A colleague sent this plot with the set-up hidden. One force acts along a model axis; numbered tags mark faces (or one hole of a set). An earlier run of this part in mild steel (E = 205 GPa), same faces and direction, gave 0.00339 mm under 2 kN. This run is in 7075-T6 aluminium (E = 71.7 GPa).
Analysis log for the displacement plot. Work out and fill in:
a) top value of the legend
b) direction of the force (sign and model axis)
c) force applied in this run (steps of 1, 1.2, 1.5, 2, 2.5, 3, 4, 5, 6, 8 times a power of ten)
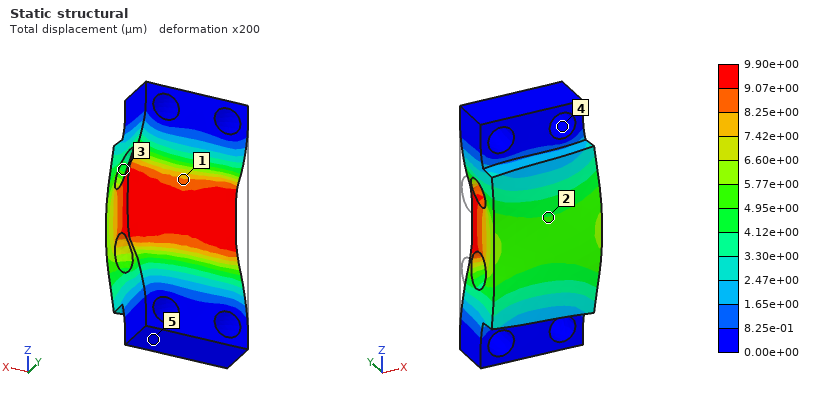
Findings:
9.90e+00 µm
+X
2 kN
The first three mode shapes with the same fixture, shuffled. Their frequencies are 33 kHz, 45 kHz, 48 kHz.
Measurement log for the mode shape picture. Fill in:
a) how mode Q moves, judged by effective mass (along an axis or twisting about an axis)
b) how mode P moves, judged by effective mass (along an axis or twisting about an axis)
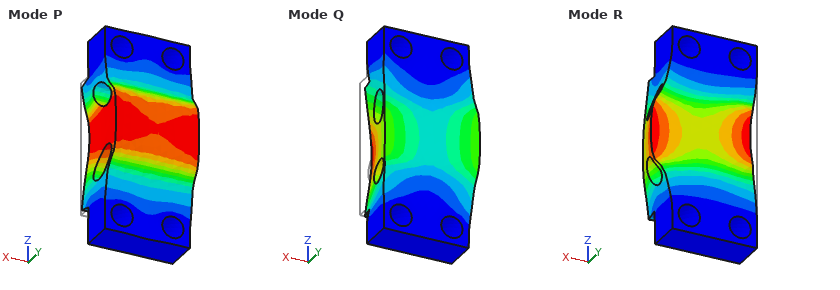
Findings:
along X
along Y
